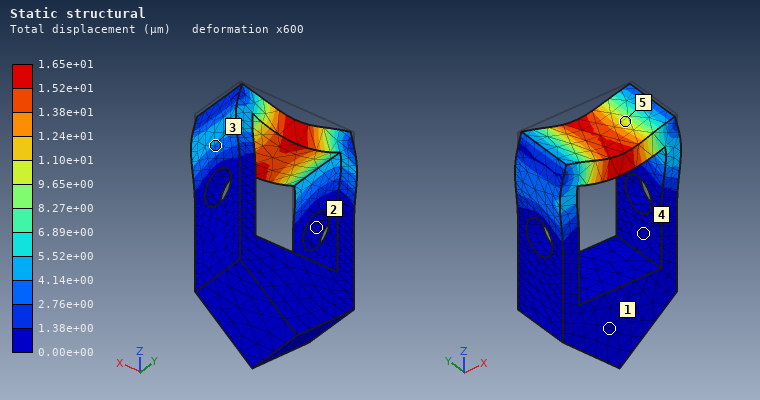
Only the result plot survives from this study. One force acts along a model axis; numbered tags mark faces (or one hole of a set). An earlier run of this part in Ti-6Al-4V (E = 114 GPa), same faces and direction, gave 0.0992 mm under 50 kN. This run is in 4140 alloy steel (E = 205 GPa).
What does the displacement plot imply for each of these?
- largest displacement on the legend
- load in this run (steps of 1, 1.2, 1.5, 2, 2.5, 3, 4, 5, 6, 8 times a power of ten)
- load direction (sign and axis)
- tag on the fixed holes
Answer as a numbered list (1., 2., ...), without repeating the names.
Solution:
1. 1.65e+01 µm
2. 15 kN
3. -Z
4. 2
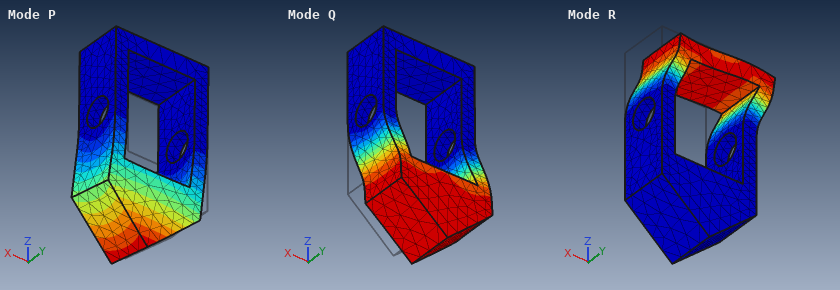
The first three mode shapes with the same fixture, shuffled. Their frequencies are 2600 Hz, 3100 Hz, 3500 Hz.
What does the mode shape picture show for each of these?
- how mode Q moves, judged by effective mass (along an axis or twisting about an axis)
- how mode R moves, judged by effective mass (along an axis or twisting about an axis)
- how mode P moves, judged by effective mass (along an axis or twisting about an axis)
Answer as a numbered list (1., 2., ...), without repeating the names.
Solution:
1. along X
2. along X
3. along Y
